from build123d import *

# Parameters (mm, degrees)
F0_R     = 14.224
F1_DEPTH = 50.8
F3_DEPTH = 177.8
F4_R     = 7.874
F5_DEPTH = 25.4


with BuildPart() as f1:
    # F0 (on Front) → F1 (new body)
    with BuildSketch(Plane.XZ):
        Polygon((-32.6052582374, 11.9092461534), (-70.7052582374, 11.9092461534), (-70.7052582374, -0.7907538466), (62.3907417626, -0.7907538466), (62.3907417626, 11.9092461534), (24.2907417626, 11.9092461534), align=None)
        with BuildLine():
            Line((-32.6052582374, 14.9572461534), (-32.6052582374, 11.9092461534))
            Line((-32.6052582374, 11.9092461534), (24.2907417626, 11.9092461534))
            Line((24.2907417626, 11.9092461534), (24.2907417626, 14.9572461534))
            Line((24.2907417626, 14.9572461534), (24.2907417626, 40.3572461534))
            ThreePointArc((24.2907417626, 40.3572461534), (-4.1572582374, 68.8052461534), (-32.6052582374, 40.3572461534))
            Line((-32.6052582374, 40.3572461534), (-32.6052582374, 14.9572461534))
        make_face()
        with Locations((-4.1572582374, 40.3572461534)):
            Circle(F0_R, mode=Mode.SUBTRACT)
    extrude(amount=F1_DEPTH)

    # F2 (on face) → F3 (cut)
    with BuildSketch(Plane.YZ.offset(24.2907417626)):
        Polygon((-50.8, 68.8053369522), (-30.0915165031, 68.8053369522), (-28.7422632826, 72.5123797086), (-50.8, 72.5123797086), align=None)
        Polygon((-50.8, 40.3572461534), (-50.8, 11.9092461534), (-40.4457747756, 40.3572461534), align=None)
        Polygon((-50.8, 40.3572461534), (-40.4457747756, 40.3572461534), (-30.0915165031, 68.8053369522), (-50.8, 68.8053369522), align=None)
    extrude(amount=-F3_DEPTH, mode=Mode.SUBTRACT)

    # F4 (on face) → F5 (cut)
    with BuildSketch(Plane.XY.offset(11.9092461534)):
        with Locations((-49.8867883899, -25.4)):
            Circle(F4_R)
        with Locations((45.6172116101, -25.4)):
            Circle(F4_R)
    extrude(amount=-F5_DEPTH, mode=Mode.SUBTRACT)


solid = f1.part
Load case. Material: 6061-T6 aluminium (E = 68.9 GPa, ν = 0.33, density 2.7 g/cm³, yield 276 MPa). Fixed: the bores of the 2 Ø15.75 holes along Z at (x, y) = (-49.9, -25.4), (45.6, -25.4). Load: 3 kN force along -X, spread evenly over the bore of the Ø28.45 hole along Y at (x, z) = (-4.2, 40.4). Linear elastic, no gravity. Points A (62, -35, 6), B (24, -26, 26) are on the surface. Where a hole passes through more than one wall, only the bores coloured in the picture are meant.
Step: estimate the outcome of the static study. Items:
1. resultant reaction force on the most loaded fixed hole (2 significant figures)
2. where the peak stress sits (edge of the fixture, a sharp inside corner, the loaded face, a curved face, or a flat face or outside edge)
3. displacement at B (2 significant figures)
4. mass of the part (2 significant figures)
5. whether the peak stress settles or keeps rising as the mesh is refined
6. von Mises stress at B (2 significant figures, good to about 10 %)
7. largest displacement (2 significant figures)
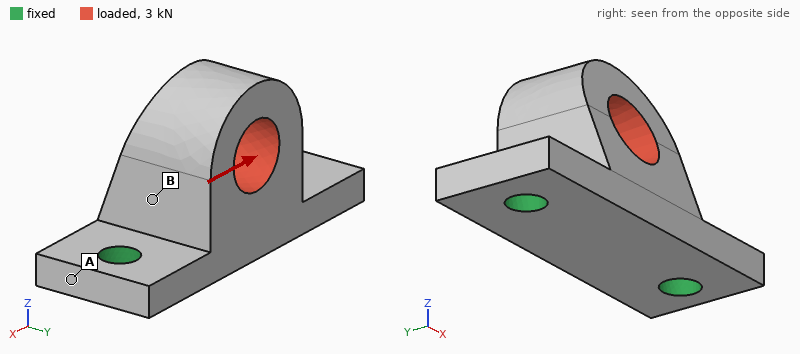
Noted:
2.1 kN
edge of the fixture
6.6 µm
470 g
keeps rising
4.5 MPa
14 µm
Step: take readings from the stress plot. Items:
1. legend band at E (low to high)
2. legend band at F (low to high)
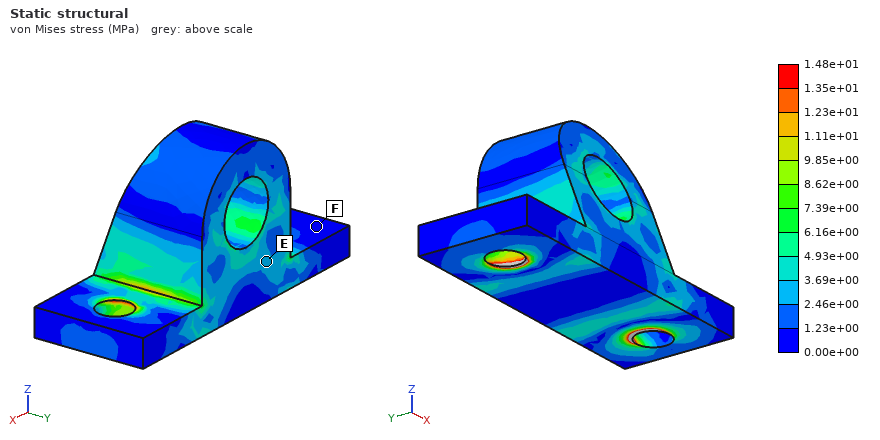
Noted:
2.46e+00 to 3.69e+00 MPa
0.00e+00 to 1.23e+00 MPa
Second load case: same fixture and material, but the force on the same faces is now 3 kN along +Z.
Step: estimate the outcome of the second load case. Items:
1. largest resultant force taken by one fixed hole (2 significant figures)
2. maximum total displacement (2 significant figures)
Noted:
1.7 kN
13 µm
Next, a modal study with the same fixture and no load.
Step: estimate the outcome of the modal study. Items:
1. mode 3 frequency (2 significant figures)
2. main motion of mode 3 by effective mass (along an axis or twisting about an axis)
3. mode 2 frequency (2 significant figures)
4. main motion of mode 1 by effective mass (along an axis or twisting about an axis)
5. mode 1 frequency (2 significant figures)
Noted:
6400 Hz
along Z
5600 Hz
along Y
2700 Hz
